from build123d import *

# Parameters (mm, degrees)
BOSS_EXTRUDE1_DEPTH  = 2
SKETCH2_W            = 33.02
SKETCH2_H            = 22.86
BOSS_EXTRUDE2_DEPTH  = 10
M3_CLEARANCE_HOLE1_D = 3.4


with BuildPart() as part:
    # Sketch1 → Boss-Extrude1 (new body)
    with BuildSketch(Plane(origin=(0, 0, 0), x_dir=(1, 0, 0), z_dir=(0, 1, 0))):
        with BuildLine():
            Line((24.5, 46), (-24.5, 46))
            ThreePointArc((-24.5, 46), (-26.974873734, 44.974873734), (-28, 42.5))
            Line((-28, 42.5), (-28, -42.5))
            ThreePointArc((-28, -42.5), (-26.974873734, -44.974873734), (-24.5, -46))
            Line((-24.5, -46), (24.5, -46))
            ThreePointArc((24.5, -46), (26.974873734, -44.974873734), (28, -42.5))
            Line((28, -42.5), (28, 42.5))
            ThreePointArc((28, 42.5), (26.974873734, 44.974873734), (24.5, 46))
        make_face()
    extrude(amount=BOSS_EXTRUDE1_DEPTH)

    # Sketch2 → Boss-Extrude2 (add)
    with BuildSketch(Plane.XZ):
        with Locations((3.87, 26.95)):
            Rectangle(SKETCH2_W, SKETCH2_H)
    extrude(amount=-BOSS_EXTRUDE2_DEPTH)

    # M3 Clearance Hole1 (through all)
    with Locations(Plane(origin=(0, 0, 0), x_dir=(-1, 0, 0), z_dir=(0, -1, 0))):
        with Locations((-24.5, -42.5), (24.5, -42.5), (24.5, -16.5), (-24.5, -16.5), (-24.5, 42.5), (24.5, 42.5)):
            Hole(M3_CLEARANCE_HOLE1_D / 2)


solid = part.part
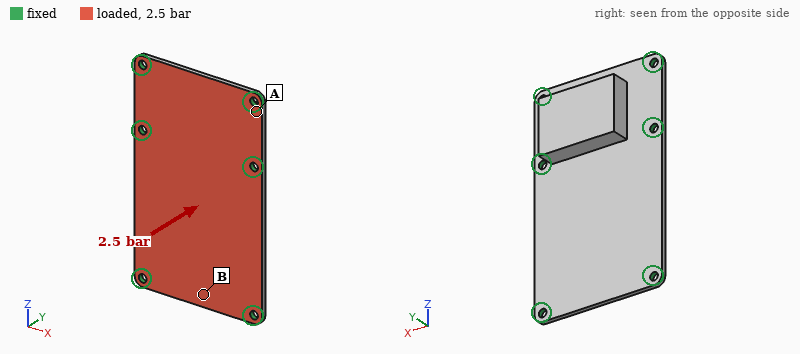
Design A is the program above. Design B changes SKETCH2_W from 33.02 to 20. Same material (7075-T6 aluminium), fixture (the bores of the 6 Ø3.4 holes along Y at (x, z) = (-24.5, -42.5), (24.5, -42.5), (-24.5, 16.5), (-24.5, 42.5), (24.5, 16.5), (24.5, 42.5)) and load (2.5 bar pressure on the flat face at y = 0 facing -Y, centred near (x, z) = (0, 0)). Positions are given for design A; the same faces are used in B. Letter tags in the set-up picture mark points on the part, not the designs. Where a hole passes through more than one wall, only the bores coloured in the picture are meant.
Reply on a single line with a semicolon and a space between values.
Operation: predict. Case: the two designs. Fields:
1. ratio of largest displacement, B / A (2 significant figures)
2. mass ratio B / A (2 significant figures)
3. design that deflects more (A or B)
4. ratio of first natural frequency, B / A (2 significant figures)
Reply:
1.1; 0.85; B; 0.95
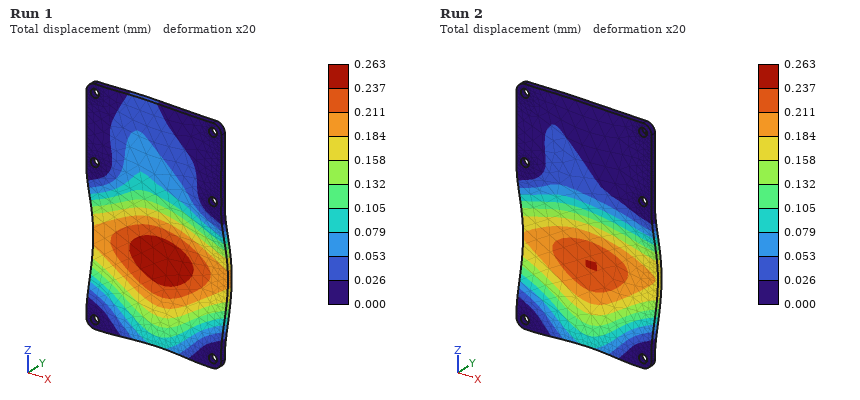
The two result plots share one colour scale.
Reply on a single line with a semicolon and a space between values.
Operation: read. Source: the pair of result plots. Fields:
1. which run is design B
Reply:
Run 1
